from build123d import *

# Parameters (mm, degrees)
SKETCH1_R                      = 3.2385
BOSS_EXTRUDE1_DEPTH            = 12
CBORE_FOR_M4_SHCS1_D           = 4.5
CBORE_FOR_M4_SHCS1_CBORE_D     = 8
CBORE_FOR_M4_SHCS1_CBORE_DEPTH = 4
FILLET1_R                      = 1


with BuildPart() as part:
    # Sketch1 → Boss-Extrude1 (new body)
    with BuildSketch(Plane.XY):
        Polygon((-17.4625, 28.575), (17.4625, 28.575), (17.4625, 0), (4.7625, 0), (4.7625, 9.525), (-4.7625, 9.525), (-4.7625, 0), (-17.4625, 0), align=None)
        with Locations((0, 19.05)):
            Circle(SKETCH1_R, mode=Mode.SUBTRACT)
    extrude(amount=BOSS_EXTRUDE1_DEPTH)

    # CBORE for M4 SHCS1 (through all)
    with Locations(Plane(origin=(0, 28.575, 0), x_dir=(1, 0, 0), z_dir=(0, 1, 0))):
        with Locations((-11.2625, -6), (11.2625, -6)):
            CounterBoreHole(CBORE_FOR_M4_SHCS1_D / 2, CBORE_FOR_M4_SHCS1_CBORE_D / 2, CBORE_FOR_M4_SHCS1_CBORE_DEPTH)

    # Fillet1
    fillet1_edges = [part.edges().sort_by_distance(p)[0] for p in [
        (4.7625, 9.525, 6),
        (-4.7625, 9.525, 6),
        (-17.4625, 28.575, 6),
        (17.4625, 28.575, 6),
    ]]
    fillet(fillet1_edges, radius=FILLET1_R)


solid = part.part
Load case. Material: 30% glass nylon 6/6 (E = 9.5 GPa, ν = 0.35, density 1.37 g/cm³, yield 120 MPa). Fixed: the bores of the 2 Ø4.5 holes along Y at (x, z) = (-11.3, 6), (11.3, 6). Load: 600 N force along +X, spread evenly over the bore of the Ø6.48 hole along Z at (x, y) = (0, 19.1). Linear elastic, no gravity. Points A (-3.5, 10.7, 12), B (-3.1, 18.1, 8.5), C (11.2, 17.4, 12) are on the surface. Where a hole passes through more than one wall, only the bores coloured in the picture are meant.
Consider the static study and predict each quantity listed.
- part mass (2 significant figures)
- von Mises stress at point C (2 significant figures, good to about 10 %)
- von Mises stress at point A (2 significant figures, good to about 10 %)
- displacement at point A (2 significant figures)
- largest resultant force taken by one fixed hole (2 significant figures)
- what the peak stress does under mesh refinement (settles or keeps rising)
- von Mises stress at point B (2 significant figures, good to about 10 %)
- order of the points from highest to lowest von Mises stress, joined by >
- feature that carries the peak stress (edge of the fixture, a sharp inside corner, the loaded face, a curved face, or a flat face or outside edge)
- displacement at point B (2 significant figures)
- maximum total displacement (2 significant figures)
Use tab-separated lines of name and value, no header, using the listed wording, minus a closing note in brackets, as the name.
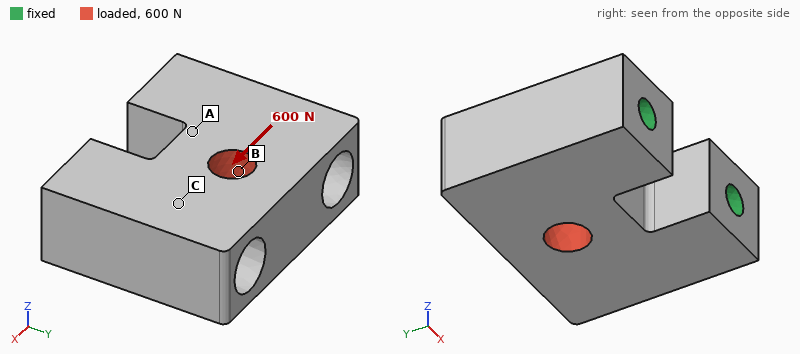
part mass	13 g
von Mises stress at point C	0.92 MPa
von Mises stress at point A	0.45 MPa
displacement at point A	0.48 µm
largest resultant force taken by one fixed hole	300 N
what the peak stress does under mesh refinement	keeps rising
von Mises stress at point B	2.6 MPa
order of the points from highest to lowest von Mises stress, joined by >	B > C > A
feature that carries the peak stress	edge of the fixture
displacement at point B	1.8 µm
maximum total displacement	2.5 µm
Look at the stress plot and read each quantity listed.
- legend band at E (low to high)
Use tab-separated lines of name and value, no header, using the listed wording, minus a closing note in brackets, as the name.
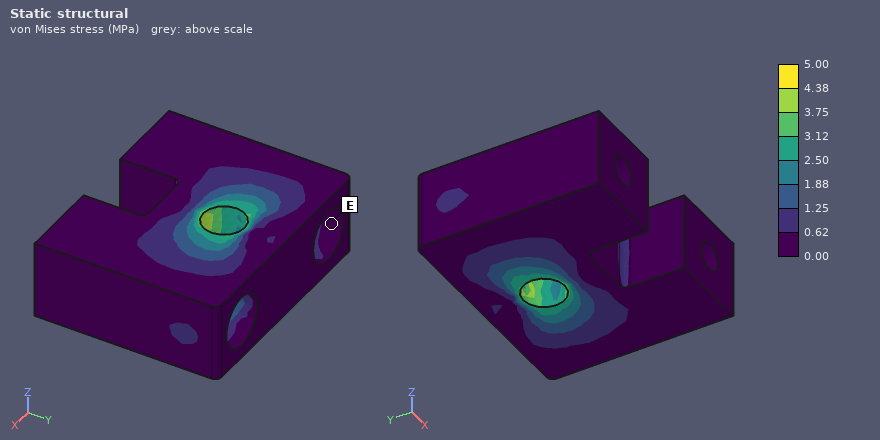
legend band at E	0.00 to 0.62 MPa
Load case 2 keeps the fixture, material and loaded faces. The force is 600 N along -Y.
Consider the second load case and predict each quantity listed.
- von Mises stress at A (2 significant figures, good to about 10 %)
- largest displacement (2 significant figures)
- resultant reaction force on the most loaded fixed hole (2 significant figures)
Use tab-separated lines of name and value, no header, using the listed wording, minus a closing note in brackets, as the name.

von Mises stress at A	2.6 MPa
largest displacement	4.9 µm
resultant reaction force on the most loaded fixed hole	310 N
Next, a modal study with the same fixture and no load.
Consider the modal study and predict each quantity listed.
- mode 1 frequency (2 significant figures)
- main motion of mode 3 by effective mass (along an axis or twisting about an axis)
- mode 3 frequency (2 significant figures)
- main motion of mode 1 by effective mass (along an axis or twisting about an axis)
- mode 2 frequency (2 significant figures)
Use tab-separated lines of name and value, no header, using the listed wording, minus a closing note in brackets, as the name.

mode 1 frequency	24 kHz
main motion of mode 3 by effective mass	along Y
mode 3 frequency	37 kHz
main motion of mode 1 by effective mass	along Z
mode 2 frequency	34 kHz
